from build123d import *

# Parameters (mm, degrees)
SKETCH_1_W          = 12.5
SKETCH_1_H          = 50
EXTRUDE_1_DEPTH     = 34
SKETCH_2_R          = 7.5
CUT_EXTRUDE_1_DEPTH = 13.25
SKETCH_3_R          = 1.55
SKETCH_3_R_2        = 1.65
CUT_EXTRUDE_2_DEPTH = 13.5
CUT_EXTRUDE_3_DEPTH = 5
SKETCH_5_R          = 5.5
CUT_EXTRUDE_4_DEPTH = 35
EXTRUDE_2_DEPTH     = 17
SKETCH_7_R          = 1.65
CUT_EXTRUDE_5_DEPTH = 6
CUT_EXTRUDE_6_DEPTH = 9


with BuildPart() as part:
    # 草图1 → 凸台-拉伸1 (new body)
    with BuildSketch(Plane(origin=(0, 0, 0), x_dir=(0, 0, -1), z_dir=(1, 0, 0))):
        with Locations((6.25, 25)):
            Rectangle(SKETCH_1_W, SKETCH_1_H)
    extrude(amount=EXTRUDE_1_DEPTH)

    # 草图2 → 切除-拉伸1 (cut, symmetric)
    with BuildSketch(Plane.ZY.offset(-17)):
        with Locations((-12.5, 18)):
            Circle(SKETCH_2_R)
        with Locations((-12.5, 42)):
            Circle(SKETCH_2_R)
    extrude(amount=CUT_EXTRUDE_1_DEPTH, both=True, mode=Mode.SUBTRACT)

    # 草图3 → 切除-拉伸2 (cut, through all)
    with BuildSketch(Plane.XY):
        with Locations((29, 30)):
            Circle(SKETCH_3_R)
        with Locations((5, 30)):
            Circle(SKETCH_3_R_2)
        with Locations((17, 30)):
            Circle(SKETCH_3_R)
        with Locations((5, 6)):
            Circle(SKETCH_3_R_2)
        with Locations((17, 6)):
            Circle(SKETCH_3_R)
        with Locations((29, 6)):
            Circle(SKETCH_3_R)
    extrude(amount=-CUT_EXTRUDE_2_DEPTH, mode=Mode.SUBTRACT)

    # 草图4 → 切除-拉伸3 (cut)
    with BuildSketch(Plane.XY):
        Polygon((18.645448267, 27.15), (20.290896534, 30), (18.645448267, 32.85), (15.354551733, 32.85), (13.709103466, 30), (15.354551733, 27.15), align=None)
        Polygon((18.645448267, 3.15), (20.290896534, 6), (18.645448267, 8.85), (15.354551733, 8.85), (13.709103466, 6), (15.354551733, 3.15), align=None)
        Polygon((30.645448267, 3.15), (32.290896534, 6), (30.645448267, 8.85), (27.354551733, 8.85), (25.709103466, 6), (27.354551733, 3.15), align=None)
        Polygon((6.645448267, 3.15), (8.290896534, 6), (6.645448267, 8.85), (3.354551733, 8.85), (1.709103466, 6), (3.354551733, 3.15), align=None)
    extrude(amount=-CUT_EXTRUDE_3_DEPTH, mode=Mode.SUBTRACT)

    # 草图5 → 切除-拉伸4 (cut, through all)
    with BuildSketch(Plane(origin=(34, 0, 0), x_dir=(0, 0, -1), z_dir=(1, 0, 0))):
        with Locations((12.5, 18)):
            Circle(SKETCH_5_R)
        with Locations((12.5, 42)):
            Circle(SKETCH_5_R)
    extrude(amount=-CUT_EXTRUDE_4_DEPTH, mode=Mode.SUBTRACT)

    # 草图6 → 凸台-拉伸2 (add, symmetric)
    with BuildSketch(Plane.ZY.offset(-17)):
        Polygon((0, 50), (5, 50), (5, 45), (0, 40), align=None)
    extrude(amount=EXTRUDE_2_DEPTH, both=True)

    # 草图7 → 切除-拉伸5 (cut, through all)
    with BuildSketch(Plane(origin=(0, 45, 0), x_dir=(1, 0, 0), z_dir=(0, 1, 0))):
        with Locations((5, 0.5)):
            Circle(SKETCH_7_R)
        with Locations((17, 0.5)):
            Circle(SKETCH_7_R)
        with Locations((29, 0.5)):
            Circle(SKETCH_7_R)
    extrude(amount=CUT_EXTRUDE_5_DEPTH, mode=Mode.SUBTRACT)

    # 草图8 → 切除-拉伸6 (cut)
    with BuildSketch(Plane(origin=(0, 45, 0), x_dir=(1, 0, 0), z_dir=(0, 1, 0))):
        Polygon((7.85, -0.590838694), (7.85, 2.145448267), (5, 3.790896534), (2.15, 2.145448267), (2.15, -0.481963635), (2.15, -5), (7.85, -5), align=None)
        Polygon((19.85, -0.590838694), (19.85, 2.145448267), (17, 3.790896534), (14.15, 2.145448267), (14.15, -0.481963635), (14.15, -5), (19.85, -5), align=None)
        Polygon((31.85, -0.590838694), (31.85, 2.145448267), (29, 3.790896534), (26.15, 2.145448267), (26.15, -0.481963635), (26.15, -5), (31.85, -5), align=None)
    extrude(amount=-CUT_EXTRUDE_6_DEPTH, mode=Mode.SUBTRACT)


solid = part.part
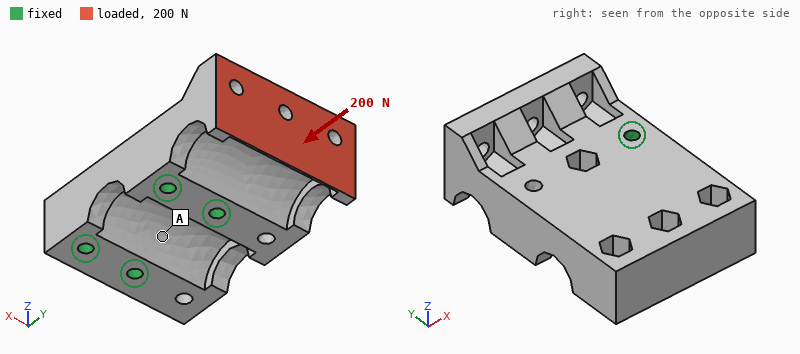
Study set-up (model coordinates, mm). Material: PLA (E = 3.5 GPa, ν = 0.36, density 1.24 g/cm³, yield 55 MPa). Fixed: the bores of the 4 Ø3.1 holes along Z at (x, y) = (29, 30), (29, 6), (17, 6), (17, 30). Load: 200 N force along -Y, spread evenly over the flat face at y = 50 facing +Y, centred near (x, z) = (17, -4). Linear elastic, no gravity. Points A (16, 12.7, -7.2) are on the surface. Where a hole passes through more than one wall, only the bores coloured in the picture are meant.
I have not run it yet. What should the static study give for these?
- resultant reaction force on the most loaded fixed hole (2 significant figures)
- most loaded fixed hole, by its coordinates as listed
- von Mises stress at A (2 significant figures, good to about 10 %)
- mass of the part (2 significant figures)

94 N
(17, 30)
0.65 MPa
19 g
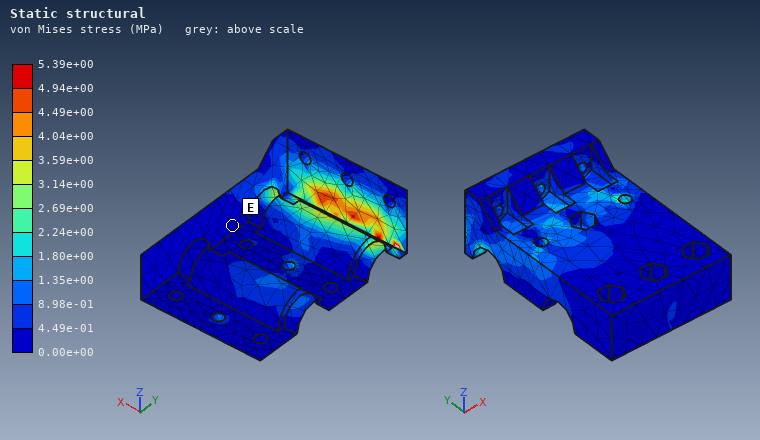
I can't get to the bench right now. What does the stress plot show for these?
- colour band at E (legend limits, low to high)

0.00e+00 to 4.49e-01 MPa
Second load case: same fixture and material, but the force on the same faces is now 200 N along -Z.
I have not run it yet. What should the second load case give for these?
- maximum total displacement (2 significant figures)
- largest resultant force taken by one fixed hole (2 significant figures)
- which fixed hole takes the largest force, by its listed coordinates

0.25 mm
240 N
(17, 30)
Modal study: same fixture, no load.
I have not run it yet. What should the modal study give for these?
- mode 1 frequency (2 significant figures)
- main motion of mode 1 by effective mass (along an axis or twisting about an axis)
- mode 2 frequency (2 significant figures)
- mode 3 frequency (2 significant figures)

3100 Hz
along Z
4600 Hz
5600 Hz
